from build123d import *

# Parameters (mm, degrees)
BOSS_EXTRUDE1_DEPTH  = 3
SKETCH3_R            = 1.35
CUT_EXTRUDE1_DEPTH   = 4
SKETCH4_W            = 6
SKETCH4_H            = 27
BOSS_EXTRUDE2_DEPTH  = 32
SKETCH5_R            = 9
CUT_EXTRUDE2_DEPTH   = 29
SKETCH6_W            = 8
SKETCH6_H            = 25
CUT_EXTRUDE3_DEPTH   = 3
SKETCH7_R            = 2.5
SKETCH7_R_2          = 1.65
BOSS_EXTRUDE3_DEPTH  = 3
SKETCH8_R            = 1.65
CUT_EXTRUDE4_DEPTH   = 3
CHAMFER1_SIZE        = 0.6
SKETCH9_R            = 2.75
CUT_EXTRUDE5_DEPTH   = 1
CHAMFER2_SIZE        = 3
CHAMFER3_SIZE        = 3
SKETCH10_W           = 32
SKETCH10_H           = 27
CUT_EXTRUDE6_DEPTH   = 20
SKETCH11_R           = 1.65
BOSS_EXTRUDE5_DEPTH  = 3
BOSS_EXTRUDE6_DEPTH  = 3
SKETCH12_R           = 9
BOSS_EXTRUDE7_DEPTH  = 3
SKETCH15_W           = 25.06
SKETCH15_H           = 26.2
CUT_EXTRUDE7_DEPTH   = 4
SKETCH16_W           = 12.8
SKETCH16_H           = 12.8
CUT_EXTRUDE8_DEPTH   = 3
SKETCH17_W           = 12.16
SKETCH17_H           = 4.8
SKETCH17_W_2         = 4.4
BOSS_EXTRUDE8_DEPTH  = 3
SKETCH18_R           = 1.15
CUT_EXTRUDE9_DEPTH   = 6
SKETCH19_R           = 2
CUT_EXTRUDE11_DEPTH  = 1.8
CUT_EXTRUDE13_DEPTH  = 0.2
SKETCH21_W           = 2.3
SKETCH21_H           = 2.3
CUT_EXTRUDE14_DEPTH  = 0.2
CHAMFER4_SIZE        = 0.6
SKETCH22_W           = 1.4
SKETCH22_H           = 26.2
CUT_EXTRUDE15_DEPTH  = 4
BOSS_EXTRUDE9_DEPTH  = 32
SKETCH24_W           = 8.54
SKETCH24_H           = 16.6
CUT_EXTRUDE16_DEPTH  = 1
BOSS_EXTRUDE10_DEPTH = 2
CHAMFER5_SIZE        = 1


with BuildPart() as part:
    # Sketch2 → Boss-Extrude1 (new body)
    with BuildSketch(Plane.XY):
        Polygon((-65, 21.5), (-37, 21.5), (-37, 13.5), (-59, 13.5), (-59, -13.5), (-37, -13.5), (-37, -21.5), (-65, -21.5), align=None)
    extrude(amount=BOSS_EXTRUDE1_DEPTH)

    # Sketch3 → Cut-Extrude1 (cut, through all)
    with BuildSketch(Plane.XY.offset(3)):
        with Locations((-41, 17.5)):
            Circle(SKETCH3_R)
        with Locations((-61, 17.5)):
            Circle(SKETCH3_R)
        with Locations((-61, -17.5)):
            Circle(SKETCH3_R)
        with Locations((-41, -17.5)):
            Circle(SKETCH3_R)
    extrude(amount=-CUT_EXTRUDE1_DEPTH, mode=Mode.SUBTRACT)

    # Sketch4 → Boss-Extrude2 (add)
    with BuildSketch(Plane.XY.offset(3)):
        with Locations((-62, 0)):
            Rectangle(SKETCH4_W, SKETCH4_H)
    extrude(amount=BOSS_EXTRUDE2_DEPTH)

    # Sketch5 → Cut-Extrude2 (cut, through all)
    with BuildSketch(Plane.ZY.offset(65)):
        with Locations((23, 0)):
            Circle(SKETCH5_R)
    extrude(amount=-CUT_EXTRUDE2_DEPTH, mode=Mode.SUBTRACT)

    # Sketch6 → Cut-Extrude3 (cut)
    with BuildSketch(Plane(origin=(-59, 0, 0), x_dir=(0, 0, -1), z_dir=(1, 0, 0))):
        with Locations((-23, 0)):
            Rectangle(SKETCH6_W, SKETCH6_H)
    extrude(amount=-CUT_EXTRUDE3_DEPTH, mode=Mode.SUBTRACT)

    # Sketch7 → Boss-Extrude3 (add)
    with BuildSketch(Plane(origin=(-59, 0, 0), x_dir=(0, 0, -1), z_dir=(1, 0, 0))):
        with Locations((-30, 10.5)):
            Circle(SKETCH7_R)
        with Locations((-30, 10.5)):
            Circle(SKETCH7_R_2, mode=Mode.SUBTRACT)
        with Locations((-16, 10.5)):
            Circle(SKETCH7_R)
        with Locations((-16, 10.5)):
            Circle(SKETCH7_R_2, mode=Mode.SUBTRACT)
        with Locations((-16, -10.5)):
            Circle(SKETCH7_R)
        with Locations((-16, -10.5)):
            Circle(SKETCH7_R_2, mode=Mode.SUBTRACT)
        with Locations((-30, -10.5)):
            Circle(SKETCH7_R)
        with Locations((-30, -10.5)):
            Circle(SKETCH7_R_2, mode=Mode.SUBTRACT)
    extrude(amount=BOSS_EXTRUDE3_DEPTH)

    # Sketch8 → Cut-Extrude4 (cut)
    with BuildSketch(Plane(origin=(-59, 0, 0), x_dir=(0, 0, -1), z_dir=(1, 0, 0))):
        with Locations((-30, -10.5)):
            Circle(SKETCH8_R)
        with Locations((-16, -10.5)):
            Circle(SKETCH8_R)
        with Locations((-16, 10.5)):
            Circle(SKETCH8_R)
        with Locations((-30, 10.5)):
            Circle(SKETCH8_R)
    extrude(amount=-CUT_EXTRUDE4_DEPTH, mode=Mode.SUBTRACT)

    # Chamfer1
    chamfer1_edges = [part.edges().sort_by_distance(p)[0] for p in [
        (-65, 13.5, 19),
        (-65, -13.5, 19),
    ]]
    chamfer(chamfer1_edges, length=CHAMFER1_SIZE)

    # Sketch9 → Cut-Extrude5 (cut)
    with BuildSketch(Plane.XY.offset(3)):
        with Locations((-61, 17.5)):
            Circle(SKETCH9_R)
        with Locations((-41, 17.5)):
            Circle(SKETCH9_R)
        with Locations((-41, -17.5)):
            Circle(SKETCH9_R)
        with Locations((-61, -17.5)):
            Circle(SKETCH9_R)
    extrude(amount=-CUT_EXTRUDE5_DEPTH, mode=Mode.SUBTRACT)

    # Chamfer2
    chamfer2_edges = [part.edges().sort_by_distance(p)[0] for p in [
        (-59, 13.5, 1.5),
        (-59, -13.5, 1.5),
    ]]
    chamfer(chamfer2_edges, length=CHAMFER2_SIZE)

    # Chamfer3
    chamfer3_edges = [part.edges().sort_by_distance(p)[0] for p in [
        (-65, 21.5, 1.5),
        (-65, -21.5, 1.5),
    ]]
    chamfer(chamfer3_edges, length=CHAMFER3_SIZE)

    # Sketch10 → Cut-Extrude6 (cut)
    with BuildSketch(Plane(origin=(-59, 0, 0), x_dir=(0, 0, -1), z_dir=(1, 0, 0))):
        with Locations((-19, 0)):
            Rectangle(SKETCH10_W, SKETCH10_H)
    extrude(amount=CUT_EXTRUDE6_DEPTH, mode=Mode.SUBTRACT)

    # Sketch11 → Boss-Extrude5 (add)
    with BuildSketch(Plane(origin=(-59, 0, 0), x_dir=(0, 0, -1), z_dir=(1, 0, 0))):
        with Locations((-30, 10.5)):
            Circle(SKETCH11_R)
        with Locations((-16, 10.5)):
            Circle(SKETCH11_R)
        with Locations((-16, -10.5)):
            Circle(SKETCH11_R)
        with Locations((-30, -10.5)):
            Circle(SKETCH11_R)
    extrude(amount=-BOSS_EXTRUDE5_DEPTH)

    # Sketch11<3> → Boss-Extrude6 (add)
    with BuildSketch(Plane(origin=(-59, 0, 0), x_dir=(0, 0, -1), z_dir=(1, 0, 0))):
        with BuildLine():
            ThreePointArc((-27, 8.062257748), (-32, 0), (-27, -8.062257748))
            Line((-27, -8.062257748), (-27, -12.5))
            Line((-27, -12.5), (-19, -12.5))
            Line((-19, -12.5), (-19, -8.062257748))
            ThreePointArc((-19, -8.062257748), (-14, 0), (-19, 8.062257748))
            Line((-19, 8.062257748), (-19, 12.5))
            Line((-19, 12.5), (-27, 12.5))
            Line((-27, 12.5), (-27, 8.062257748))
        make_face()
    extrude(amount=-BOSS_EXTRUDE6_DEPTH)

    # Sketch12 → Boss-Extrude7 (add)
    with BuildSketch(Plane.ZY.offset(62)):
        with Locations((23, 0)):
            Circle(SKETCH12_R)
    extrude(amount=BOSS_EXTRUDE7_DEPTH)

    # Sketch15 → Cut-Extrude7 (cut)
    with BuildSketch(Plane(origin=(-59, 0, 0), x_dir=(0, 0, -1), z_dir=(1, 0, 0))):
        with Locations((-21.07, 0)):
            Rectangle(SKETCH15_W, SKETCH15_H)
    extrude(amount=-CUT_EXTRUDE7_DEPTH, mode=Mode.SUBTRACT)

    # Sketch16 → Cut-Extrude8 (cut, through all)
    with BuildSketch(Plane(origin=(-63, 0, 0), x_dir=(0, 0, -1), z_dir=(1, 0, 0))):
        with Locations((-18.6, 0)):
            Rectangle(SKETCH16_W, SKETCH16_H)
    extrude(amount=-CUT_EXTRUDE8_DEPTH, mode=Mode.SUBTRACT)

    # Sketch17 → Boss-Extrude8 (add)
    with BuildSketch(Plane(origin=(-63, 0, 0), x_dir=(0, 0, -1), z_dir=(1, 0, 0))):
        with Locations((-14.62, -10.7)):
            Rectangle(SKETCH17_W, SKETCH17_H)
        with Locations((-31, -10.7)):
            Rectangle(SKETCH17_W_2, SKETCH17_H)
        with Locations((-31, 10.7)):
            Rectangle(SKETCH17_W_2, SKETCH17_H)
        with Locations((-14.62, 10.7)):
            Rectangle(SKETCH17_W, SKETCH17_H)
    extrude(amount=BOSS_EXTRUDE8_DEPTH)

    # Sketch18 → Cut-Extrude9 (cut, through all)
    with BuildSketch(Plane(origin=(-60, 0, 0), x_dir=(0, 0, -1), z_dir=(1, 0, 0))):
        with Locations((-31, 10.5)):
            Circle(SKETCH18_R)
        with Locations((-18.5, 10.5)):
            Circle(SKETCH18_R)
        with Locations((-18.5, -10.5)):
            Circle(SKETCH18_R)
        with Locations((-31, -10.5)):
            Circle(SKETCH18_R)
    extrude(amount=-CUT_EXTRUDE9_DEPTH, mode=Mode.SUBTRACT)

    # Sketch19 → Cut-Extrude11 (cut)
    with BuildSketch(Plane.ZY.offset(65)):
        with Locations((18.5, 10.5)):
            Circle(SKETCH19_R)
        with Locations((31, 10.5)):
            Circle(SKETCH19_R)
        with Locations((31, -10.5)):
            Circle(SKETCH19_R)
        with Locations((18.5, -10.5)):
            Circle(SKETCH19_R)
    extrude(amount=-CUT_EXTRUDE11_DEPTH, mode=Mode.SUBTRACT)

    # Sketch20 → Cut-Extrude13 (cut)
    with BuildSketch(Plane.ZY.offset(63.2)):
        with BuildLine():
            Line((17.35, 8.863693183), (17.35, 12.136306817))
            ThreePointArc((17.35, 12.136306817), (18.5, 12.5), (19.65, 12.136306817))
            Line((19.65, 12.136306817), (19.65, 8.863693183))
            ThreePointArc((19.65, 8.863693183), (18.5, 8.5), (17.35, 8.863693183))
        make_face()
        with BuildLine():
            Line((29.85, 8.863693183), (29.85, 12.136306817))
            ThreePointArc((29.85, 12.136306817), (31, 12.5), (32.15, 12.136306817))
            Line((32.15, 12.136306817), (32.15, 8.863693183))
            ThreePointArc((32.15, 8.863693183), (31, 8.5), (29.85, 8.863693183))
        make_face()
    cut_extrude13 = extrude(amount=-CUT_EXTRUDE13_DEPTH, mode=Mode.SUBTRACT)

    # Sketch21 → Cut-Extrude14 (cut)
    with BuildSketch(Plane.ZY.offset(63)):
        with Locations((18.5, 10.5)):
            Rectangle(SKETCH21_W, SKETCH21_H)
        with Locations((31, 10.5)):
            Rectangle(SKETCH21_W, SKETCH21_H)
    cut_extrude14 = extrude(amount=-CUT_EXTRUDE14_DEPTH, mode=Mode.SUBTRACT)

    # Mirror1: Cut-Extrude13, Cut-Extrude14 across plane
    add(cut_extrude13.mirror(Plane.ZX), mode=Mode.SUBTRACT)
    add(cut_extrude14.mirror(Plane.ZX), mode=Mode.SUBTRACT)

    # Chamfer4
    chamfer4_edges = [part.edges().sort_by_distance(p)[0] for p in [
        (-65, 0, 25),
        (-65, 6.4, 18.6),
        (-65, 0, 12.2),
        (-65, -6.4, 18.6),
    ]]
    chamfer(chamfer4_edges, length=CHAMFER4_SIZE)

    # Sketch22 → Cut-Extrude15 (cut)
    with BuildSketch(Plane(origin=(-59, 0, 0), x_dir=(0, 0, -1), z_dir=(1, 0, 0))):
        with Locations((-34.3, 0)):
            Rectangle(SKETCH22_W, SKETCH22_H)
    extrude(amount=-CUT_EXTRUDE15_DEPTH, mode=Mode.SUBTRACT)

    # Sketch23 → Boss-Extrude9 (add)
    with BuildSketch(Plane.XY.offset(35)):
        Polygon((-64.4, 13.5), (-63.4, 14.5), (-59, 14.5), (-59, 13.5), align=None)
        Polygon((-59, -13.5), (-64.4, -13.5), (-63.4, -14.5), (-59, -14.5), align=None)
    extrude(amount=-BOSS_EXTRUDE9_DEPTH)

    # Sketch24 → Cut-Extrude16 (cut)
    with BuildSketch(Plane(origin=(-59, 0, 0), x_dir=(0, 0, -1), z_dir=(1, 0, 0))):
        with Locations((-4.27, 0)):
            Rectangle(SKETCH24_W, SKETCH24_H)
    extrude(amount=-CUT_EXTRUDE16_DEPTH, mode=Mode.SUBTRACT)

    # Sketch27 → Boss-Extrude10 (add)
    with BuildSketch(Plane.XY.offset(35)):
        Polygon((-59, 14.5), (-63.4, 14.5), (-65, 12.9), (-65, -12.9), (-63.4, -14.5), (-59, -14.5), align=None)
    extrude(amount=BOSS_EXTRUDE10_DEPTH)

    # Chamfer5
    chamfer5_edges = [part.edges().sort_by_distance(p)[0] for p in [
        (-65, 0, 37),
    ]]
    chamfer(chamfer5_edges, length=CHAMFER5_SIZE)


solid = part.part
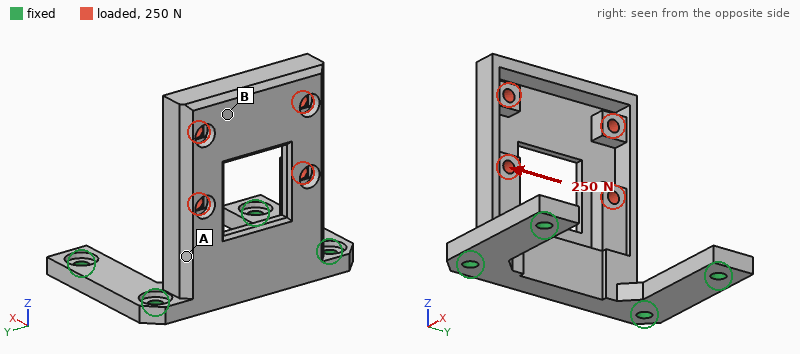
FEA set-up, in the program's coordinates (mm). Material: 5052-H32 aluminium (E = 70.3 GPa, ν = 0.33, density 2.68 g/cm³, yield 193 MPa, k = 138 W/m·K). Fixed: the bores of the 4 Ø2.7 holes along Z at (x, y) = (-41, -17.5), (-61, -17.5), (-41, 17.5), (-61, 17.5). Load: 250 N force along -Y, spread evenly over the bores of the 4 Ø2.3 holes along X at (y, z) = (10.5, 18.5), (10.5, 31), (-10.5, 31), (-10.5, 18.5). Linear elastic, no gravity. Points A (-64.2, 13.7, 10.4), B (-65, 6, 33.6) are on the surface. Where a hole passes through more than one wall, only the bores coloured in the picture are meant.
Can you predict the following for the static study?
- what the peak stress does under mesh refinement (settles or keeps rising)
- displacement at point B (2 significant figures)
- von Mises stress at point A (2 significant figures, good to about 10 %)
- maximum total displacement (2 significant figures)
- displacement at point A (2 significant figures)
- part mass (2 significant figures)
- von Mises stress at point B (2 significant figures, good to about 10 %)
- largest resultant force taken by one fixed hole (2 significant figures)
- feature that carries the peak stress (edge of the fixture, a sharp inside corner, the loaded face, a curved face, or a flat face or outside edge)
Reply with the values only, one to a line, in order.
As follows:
keeps rising
29 µm
27 MPa
56 µm
9.6 µm
12 g
6.2 MPa
230 N
edge of the fixture
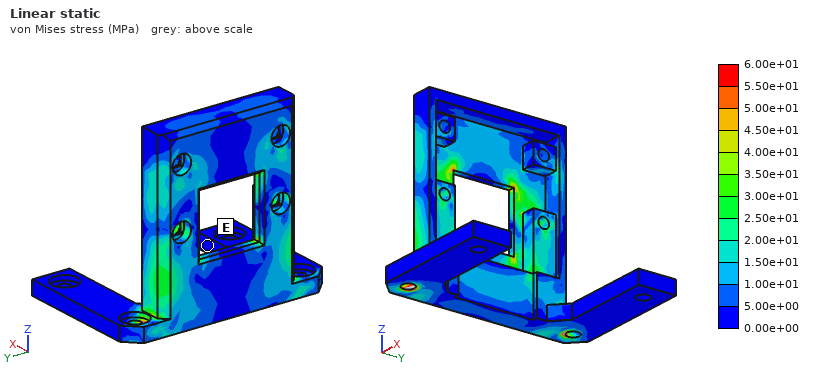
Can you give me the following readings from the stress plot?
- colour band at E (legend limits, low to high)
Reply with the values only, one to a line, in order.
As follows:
0.00e+00 to 5.00e+00 MPa
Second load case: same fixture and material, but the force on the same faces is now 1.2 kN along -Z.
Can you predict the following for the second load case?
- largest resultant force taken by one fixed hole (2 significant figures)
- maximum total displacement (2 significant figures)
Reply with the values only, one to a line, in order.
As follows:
660 N
47 µm
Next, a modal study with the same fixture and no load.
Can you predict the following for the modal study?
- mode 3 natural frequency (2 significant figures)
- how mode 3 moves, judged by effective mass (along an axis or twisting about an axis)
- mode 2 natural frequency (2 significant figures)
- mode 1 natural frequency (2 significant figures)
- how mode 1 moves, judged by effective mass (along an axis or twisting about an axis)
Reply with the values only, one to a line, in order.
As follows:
8200 Hz
along Y
4600 Hz
1900 Hz
along X
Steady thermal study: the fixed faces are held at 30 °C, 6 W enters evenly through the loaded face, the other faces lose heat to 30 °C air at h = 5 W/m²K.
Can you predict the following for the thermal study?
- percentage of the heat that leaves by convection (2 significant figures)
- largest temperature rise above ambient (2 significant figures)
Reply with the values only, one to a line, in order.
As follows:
3.6 %
22 K
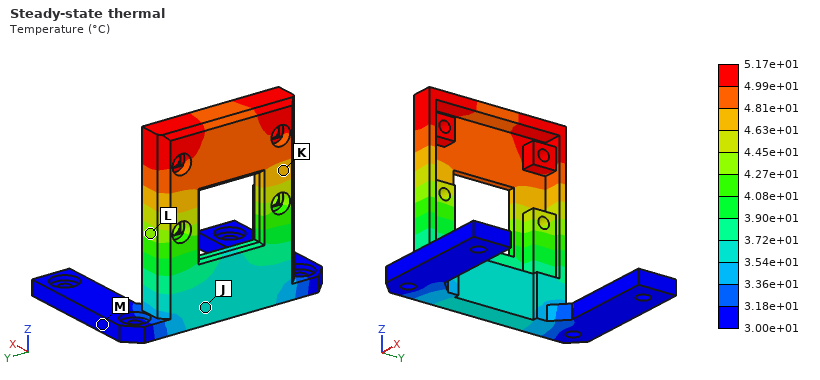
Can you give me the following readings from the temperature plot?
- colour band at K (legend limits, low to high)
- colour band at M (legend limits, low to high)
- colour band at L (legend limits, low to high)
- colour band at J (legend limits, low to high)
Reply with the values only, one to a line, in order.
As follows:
4.63e+01 to 4.81e+01 °C
3.00e+01 to 3.18e+01 °C
4.27e+01 to 4.45e+01 °C
3.54e+01 to 3.72e+01 °C
